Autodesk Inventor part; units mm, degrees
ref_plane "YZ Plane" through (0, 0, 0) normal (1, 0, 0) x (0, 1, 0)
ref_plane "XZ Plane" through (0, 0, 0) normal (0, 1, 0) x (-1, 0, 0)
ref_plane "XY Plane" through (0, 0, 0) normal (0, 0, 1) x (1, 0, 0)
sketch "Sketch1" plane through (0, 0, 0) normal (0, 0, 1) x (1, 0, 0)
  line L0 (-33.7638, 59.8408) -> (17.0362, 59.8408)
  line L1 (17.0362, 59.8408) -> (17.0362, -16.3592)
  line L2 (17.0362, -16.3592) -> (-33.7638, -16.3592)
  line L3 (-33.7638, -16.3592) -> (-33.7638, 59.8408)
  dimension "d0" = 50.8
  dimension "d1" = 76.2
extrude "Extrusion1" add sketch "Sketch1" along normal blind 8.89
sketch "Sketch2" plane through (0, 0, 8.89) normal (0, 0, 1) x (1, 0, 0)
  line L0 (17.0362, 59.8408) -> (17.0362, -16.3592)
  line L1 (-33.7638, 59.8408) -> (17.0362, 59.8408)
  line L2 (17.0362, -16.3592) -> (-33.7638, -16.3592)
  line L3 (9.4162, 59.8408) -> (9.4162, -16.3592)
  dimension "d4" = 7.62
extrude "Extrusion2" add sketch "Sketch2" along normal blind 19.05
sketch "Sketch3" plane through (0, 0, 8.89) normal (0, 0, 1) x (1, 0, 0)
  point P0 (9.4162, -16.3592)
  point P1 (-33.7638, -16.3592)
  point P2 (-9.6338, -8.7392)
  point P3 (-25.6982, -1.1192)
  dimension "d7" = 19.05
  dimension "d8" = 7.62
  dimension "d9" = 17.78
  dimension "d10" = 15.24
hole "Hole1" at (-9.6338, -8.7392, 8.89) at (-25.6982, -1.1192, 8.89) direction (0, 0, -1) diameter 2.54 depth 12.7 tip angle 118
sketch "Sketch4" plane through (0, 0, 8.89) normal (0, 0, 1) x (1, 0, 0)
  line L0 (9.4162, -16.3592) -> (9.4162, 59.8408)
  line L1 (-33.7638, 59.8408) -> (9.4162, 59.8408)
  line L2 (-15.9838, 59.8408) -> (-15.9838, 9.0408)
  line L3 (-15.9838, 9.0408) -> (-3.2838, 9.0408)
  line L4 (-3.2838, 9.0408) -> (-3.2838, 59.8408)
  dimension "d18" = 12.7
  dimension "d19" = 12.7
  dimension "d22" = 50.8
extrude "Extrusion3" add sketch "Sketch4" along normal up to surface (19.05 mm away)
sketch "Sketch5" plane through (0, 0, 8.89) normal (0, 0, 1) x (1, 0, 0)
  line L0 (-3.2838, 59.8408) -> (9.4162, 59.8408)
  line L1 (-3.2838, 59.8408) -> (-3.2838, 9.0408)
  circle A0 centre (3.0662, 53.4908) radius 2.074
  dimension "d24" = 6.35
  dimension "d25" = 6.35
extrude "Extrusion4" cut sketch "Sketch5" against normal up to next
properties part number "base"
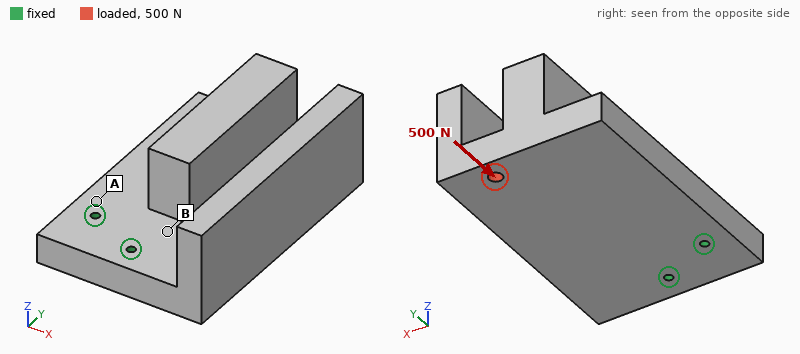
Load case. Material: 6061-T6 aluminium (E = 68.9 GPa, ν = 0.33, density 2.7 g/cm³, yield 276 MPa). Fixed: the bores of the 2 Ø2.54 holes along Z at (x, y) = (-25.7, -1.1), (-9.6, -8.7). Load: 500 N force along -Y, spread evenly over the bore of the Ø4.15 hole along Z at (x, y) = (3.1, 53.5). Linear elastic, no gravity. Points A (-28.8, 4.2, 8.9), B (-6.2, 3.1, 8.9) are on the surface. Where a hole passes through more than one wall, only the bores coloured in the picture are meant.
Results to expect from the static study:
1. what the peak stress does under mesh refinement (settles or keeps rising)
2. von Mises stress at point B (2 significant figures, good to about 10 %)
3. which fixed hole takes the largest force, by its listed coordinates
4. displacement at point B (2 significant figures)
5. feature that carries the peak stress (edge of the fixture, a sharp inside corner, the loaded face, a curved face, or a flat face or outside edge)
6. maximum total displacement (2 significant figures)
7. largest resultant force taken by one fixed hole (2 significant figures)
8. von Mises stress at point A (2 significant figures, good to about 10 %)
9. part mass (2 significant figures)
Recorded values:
keeps rising
4.1 MPa
(-9.6, -8.7)
1.7 µm
edge of the fixture
9.5 µm
770 N
1.7 MPa
160 g
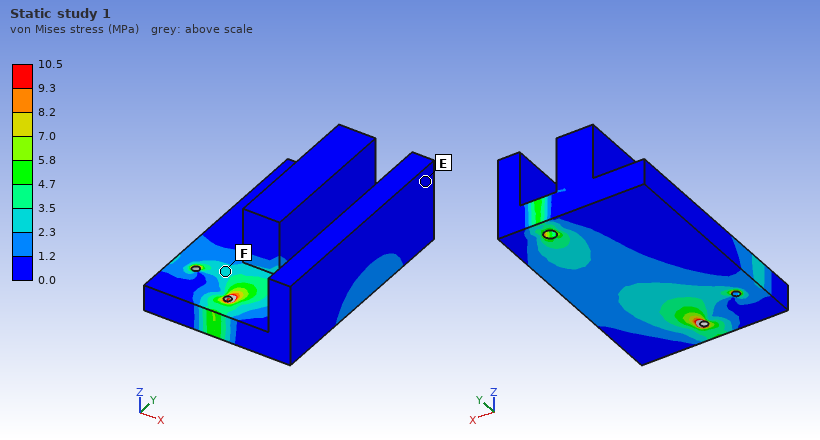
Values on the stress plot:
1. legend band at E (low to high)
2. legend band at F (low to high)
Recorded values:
0.0 to 1.2 MPa
2.3 to 3.5 MPa
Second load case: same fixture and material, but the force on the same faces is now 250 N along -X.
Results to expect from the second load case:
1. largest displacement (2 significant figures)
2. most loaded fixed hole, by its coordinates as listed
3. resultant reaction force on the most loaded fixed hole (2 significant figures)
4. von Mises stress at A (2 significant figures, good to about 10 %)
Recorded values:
13 µm
(-25.7, -1.1)
820 N
4.3 MPa
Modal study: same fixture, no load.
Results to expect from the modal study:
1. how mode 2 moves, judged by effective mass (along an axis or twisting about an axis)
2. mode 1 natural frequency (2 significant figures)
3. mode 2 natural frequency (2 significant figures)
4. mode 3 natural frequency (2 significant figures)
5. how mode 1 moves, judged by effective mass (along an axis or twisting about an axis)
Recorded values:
along X
1100 Hz
2600 Hz
3400 Hz
along Z
